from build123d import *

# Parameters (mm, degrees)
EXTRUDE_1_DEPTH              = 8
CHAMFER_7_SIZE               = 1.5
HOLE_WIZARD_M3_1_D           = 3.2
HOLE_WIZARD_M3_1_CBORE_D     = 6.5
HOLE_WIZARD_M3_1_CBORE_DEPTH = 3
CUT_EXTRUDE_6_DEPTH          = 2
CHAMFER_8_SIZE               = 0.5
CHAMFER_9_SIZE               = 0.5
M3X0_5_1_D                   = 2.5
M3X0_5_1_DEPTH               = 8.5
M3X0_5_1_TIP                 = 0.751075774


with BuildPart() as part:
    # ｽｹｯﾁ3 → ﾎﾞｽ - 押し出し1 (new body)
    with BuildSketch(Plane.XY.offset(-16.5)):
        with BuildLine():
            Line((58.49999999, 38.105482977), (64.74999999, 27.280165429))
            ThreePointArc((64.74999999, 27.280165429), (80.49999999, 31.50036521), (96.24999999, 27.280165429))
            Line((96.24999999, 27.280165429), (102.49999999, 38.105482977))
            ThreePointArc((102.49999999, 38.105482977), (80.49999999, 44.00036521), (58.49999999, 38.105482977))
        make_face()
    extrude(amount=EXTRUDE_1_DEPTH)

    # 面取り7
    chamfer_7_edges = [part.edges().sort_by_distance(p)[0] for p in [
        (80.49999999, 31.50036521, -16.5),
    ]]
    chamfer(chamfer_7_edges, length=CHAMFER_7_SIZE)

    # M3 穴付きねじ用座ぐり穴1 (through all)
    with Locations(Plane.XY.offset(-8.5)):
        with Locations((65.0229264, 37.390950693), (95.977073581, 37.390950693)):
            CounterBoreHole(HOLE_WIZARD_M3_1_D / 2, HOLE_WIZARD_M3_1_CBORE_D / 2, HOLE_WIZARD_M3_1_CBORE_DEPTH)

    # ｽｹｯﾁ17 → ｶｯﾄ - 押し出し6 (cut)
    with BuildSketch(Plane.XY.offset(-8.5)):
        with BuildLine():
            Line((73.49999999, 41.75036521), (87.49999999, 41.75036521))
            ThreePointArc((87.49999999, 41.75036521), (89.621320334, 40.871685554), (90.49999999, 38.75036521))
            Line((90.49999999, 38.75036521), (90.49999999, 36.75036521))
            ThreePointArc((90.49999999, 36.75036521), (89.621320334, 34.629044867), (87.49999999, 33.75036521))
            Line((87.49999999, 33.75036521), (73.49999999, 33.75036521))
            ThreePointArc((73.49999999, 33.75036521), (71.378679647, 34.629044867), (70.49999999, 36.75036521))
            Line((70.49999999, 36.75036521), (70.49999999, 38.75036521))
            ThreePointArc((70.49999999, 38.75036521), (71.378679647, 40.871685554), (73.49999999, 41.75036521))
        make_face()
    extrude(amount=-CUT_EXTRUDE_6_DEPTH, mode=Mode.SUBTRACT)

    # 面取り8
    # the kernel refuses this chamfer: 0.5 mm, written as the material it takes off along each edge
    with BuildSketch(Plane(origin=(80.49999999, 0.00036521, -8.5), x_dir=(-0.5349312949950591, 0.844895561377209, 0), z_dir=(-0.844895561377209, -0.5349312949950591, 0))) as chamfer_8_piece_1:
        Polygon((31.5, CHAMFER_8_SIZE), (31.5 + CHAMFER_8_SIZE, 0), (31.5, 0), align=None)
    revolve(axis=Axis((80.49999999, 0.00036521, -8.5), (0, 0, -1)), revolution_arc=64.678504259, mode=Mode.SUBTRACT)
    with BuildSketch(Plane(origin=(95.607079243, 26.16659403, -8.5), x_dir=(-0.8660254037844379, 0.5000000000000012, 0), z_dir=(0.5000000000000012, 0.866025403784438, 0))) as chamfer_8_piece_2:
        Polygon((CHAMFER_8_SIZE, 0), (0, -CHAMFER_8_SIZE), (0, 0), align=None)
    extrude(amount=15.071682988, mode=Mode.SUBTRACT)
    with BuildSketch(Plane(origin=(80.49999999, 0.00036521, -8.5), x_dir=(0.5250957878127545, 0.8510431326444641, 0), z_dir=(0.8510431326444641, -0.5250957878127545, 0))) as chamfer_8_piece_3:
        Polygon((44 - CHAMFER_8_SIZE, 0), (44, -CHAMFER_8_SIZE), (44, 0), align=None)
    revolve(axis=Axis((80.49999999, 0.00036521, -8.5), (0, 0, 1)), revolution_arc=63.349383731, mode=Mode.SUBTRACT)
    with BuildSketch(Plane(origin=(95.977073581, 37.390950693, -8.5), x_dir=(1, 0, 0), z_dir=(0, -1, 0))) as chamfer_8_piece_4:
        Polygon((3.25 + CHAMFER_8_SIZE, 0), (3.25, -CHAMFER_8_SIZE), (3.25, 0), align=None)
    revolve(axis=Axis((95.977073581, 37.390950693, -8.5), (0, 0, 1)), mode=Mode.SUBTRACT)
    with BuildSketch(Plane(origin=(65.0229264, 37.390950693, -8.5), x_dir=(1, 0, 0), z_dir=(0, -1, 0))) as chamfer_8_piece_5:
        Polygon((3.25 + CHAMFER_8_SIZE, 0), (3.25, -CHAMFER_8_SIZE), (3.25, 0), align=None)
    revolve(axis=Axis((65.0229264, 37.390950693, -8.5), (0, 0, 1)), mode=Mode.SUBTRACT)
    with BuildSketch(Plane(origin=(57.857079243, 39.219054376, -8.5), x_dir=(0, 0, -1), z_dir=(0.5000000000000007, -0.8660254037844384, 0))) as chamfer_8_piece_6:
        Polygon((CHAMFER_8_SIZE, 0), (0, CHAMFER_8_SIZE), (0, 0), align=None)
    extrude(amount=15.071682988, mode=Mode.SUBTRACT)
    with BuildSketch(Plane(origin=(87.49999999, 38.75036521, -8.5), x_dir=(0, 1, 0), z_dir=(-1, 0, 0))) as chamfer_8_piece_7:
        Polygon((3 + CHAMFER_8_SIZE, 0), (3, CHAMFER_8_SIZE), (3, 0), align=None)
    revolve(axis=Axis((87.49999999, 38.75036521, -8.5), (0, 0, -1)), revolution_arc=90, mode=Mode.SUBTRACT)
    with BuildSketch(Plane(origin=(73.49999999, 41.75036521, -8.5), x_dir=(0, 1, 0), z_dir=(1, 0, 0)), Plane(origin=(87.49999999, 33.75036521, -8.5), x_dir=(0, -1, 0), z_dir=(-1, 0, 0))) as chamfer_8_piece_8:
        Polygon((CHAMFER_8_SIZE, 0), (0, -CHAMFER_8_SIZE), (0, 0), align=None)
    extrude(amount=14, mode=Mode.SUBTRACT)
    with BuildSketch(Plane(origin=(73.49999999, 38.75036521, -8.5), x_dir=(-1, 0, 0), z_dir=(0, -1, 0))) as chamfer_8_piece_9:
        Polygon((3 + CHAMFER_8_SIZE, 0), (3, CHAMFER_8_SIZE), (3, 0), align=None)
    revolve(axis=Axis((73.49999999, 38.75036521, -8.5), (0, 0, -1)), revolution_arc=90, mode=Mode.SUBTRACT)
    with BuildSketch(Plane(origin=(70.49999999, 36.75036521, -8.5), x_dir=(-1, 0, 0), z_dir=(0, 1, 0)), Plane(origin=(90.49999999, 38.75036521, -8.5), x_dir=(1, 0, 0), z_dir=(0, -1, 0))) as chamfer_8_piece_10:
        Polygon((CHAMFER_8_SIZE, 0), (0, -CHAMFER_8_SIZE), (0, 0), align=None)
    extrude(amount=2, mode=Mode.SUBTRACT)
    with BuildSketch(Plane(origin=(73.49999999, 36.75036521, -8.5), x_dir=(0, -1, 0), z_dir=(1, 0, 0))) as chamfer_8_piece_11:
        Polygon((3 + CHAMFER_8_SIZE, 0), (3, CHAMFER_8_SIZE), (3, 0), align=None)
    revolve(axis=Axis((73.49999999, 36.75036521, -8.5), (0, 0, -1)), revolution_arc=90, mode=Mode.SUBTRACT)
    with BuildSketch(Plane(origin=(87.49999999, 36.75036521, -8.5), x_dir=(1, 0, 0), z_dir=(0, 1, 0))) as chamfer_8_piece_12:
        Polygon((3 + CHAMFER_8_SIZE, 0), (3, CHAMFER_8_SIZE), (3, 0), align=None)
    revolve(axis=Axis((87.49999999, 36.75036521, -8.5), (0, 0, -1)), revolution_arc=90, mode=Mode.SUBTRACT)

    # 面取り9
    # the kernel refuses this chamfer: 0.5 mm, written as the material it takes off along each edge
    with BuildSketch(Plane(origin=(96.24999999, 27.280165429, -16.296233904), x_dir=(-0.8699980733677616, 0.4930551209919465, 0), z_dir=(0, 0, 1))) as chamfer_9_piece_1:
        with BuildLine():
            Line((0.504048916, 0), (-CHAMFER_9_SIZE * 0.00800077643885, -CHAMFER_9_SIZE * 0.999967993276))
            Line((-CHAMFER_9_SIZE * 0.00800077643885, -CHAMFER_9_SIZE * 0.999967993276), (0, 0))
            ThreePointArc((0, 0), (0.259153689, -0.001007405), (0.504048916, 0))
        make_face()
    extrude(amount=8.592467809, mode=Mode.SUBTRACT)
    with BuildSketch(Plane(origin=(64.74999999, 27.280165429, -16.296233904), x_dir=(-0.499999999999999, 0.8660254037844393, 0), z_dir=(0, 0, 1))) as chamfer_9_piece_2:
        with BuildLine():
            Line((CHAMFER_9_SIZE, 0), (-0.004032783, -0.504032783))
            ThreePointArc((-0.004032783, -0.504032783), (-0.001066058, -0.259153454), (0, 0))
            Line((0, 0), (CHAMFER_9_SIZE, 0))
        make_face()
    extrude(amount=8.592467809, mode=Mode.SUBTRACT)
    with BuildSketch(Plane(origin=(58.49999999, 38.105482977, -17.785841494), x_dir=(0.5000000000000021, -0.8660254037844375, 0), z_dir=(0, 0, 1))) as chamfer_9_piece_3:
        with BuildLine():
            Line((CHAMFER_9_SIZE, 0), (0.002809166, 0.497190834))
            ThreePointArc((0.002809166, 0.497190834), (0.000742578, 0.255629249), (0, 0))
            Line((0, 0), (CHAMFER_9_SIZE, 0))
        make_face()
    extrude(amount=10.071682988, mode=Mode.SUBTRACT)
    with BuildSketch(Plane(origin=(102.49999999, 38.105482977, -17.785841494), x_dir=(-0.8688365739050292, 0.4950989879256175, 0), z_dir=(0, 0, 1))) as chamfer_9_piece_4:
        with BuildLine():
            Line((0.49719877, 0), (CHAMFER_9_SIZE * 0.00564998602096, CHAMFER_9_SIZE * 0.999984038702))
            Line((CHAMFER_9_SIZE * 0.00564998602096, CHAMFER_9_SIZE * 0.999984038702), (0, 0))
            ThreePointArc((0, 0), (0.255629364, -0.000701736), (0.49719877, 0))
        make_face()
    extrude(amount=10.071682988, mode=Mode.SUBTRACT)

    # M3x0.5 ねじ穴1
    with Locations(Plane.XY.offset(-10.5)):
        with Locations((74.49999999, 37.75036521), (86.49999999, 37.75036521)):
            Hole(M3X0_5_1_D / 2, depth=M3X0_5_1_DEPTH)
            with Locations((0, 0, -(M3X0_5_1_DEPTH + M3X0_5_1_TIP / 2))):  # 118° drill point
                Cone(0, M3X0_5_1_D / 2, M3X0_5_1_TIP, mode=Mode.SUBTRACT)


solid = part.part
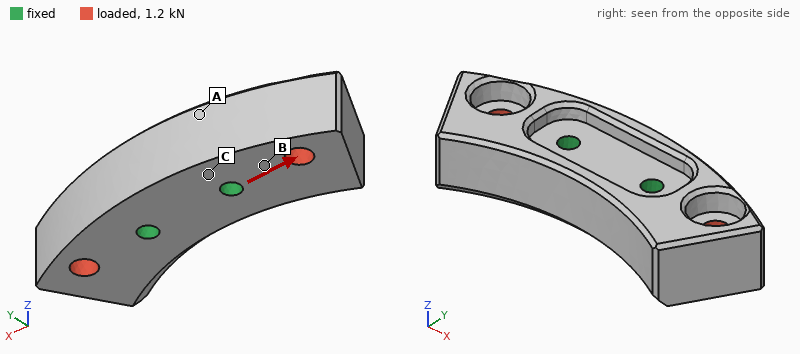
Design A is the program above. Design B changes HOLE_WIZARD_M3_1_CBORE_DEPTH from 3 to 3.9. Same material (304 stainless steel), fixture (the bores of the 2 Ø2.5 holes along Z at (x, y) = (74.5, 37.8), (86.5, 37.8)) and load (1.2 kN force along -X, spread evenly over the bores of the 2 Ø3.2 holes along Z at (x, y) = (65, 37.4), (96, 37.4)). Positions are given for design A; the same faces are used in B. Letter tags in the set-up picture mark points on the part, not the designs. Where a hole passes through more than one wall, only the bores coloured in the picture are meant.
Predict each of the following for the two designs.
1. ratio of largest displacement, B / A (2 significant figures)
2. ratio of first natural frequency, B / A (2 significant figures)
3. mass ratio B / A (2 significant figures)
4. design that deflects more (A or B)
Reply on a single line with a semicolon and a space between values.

1.4; 1.0; 0.99; B
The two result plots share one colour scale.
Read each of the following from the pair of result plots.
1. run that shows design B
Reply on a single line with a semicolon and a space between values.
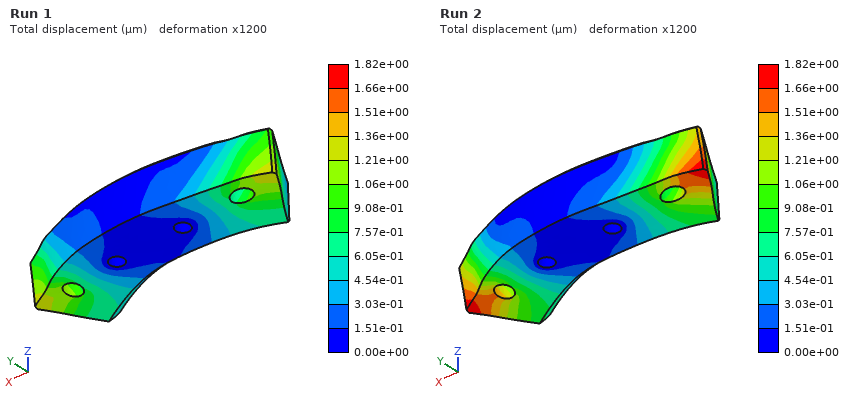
Run 2
